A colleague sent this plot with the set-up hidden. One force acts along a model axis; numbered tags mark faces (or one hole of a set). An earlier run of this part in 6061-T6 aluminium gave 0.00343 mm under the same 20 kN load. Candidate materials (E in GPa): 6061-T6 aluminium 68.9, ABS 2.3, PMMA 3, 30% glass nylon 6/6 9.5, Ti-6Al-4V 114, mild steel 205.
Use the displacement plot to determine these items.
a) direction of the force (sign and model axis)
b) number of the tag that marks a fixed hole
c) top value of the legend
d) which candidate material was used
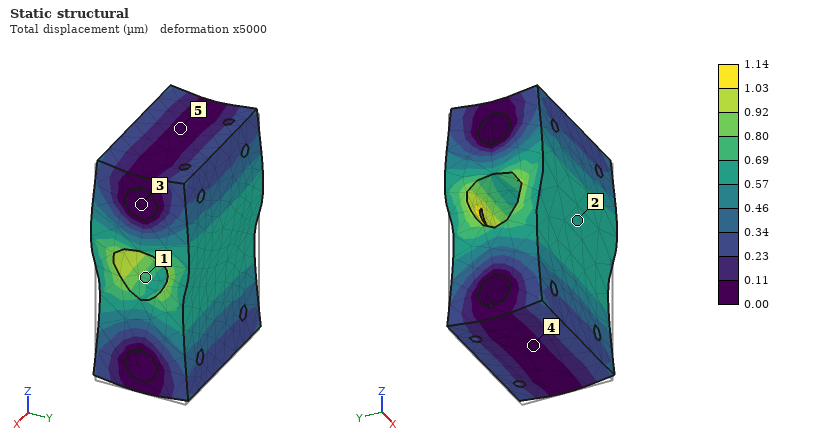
+Z
3
1.14 µm
mild steel
